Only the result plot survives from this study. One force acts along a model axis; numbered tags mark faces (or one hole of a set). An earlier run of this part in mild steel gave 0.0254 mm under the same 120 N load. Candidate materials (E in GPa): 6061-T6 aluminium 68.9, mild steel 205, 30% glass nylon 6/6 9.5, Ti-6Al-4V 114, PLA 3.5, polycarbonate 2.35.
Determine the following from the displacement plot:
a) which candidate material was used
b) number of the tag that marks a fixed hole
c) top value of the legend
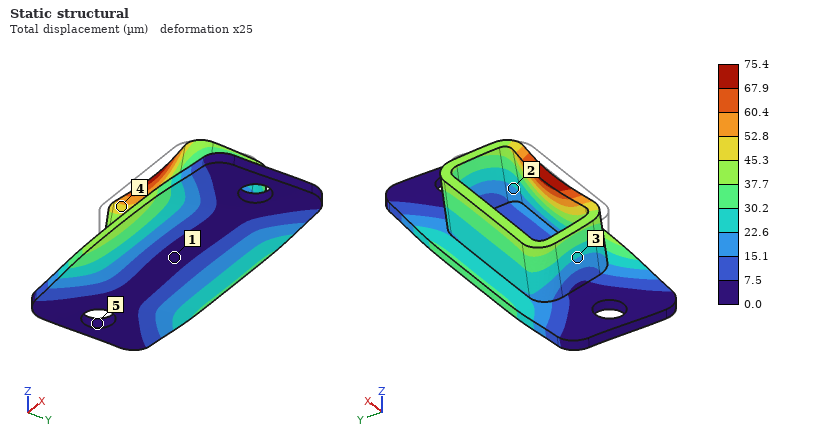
6061-T6 aluminium
5
75.4 µm
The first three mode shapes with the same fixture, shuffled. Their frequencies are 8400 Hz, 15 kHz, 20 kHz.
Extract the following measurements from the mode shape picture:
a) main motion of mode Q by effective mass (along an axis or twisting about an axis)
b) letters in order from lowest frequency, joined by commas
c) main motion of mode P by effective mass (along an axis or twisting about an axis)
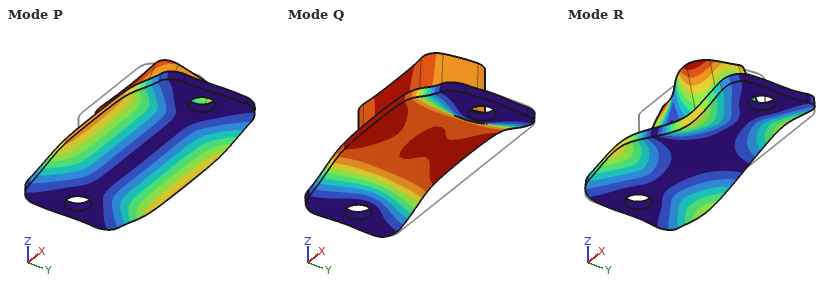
along Z
P, Q, R
along Y
